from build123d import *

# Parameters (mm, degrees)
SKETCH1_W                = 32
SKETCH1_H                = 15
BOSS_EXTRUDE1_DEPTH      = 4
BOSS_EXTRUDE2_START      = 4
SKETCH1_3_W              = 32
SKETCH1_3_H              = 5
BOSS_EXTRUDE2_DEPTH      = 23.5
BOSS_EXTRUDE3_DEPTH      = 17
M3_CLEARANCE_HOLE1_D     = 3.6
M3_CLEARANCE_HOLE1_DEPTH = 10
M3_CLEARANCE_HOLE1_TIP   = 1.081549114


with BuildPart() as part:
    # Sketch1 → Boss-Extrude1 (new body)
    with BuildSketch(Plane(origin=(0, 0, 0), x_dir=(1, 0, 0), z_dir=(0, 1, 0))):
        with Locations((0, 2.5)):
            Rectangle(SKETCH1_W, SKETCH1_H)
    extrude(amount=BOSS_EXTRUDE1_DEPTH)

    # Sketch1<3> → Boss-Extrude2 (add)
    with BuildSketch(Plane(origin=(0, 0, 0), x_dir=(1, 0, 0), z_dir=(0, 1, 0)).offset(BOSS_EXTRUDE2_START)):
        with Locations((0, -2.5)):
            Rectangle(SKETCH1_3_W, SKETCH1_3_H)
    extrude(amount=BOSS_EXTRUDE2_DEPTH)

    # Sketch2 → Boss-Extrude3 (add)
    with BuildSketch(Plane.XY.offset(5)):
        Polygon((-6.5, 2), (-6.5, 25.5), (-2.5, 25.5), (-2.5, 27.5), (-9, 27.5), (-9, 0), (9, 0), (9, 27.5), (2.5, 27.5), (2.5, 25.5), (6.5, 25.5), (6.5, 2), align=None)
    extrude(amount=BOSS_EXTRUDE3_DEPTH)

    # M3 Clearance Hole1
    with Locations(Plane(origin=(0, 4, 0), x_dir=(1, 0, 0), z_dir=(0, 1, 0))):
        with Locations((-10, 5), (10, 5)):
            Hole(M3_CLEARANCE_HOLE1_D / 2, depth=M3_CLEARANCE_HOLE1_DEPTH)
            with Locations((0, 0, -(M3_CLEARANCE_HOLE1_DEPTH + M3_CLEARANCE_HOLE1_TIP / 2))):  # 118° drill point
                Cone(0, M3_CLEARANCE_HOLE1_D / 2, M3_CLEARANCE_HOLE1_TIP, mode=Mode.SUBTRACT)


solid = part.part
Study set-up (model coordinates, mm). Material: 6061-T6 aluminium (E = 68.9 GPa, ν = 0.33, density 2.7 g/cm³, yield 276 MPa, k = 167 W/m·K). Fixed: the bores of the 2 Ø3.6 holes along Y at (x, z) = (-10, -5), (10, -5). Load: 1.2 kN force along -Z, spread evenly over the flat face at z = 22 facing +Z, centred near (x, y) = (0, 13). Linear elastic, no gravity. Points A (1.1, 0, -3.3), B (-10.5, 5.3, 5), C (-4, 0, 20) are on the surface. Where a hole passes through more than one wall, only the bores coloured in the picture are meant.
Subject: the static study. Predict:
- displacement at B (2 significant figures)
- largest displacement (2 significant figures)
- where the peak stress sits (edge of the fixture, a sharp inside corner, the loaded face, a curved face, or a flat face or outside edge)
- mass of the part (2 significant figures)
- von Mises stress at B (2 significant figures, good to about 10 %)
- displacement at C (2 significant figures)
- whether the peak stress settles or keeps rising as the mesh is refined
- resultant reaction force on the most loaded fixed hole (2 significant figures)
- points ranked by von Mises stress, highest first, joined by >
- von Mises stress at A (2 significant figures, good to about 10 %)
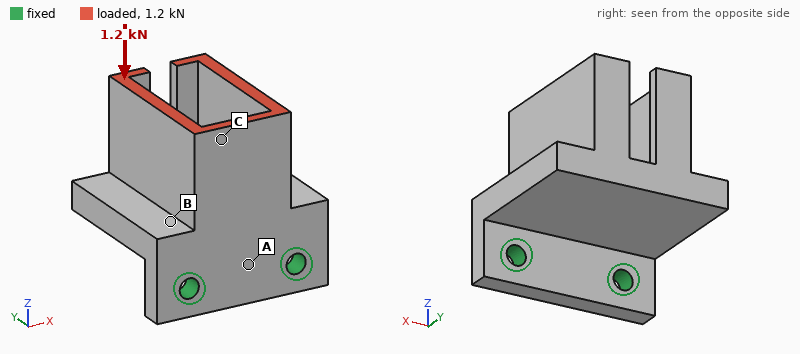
0.058 mm
0.30 mm
edge of the fixture
23 g
42 MPa
0.18 mm
keeps rising
610 N
A > B > C
75 MPa
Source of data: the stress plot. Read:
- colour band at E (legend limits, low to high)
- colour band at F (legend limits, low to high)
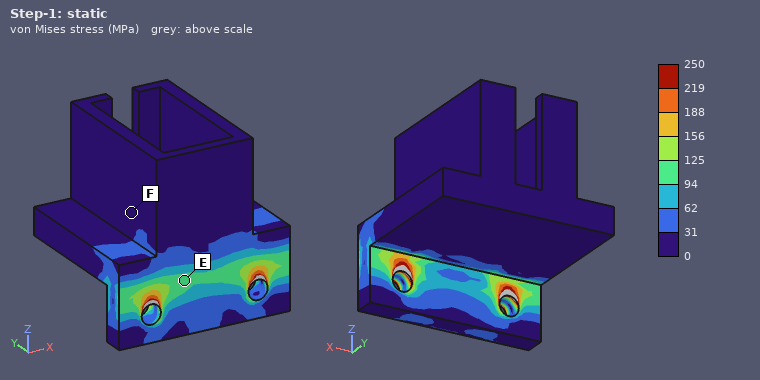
94 to 125 MPa
0 to 31 MPa
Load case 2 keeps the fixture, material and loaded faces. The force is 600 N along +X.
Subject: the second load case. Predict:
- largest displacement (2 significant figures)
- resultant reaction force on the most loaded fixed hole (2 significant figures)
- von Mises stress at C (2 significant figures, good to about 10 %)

86 µm
850 N
42 MPa
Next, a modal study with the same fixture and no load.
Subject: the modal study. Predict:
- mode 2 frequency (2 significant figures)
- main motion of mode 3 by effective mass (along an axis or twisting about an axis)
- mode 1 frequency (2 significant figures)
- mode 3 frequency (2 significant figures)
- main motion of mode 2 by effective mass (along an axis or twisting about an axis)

7300 Hz
along X
2500 Hz
7700 Hz
along X
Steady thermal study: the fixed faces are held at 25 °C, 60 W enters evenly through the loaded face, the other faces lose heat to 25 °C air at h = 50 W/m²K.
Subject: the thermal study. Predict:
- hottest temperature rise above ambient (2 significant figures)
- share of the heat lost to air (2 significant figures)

64 K
15 %
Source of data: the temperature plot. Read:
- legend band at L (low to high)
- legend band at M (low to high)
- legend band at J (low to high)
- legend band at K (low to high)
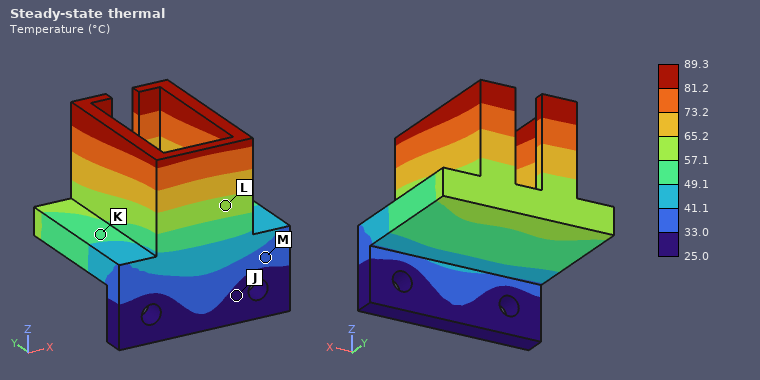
57.1 to 65.2 °C
33.0 to 41.1 °C
25.0 to 33.0 °C
49.1 to 57.1 °C
